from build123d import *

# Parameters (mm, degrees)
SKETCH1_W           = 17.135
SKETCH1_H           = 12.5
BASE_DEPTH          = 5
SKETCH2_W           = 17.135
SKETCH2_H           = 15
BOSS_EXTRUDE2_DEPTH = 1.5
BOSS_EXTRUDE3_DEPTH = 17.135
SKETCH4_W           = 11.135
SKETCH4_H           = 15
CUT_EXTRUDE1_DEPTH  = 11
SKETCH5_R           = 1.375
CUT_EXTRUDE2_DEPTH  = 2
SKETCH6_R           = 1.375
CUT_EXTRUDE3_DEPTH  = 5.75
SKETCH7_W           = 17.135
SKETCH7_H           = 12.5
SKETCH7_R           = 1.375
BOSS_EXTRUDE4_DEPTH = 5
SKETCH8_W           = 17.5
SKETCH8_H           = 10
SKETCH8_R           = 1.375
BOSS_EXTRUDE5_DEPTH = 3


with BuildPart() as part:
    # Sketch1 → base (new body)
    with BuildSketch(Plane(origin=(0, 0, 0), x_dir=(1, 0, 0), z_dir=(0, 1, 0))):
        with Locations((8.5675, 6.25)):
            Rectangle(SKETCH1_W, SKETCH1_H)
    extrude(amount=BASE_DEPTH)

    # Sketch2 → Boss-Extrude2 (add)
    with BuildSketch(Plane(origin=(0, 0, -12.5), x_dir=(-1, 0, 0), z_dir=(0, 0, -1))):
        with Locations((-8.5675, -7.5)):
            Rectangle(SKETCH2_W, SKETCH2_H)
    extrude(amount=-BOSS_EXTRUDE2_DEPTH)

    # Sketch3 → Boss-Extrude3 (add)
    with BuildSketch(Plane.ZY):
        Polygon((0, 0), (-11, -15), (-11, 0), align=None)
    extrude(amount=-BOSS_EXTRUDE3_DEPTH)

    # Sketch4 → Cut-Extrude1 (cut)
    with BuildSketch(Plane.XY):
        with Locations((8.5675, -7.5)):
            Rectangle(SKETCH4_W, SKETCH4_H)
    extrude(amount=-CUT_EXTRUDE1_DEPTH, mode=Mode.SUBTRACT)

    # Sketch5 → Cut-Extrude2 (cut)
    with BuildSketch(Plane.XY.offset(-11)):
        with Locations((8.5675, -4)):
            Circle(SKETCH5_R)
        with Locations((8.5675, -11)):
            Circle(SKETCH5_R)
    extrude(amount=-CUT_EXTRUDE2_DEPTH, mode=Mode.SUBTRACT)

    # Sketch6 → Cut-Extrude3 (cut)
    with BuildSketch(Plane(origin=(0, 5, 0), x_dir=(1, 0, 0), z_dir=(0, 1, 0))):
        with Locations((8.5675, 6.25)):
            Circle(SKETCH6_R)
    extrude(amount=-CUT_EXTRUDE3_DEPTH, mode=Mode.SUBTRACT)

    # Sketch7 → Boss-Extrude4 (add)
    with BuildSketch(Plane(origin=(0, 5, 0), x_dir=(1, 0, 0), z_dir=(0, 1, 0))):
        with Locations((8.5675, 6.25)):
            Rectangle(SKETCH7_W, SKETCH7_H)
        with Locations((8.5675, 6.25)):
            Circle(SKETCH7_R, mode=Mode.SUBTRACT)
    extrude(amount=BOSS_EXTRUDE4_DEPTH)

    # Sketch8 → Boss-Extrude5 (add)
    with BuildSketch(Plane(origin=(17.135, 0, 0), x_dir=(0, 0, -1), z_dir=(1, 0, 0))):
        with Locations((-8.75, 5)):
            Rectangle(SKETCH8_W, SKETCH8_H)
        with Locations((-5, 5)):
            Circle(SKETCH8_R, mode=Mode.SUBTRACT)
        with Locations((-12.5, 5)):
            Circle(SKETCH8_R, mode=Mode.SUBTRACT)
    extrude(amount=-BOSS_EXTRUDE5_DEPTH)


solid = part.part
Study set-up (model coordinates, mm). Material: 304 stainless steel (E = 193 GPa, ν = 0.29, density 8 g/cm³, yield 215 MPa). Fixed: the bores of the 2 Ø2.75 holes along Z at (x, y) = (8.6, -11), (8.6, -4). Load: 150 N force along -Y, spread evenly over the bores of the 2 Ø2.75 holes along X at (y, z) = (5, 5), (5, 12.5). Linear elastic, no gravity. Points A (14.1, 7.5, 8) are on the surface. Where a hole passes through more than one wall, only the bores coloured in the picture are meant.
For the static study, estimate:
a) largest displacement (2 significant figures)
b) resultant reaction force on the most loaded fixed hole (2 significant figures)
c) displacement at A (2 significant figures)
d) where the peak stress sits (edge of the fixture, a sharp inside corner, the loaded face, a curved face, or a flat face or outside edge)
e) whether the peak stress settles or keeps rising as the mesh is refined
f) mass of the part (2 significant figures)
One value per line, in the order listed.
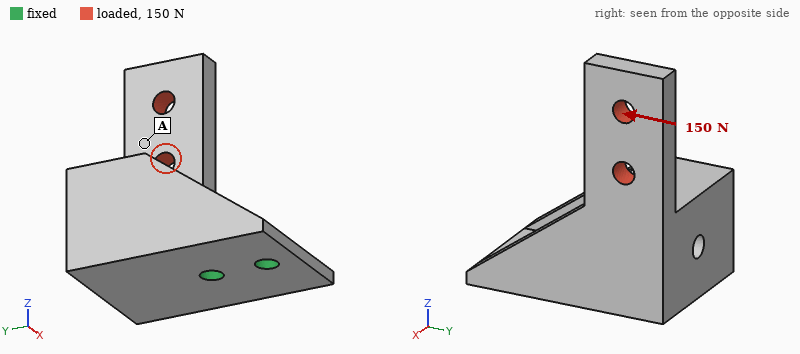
57 µm
340 N
39 µm
edge of the fixture
keeps rising
27 g
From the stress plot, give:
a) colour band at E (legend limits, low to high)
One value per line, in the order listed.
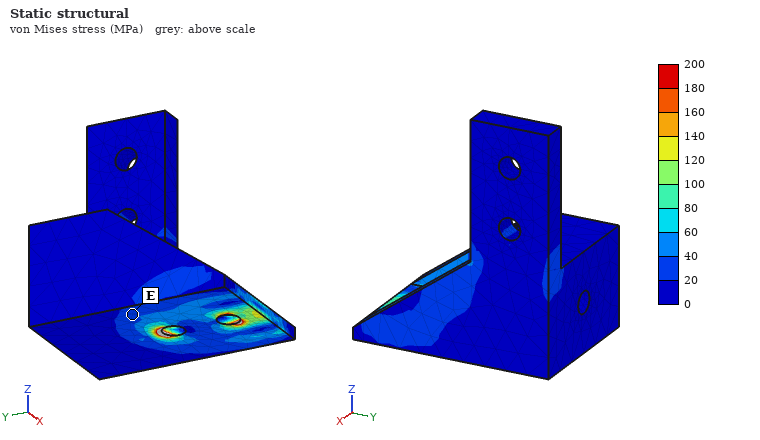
20 to 40 MPa
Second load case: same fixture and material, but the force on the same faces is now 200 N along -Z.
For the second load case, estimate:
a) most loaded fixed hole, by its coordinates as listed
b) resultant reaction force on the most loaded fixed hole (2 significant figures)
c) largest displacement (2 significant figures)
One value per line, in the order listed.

(8.6, -4)
340 N
57 µm
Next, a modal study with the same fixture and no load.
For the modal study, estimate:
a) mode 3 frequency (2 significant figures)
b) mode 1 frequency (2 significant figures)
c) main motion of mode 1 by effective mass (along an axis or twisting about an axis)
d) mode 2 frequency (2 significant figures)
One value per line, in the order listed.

8600 Hz
2600 Hz
along X
3300 Hz
